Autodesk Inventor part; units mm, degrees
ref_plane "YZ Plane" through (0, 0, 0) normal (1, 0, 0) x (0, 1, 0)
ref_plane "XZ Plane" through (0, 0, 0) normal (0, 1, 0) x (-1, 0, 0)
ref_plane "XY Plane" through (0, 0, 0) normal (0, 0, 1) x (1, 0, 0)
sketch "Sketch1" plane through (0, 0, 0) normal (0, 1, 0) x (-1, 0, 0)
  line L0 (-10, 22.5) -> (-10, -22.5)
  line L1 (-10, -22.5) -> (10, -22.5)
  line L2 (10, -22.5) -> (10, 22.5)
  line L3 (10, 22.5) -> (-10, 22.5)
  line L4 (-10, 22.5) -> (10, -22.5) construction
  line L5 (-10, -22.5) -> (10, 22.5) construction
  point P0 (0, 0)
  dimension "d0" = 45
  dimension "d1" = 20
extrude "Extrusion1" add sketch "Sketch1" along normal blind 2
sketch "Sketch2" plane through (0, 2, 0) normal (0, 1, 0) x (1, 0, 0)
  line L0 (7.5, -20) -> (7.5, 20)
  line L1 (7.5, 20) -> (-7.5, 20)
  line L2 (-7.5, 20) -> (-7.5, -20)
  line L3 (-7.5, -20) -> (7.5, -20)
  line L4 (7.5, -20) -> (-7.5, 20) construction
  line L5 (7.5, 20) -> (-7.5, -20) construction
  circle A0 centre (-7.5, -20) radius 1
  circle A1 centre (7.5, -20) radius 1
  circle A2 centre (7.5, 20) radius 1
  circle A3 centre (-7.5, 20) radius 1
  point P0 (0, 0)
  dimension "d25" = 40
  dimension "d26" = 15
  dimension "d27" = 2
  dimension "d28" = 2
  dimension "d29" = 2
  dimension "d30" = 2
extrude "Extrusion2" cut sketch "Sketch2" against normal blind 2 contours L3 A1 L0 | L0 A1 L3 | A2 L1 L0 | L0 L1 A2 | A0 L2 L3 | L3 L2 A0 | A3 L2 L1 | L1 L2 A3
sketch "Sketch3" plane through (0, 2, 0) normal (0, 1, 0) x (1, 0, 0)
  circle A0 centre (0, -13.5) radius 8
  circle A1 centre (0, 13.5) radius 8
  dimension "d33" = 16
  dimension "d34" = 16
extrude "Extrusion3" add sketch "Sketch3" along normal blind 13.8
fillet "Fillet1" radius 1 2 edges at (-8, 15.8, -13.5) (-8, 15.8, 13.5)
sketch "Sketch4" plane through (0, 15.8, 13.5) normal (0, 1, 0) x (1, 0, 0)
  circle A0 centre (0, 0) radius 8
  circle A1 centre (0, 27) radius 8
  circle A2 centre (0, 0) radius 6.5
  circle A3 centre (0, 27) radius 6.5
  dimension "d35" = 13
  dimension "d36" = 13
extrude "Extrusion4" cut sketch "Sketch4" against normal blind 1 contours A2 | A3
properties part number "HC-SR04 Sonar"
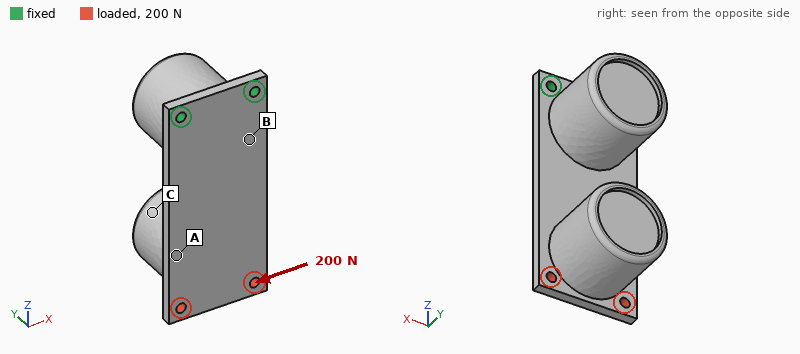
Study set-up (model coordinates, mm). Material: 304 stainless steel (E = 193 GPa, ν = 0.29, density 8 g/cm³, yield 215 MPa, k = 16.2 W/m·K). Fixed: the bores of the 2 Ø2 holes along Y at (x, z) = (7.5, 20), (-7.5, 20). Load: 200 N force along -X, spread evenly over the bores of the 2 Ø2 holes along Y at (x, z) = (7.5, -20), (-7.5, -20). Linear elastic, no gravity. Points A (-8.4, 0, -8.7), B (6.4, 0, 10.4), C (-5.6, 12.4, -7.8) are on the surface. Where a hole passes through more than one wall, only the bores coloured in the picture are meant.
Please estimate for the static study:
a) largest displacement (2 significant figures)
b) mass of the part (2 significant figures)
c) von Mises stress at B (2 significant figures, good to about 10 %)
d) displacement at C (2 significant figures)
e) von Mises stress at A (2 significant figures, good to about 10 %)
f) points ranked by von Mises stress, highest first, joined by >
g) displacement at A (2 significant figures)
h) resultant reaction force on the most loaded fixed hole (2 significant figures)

20 µm
56 g
24 MPa
9.4 µm
14 MPa
B > A > C
12 µm
530 N
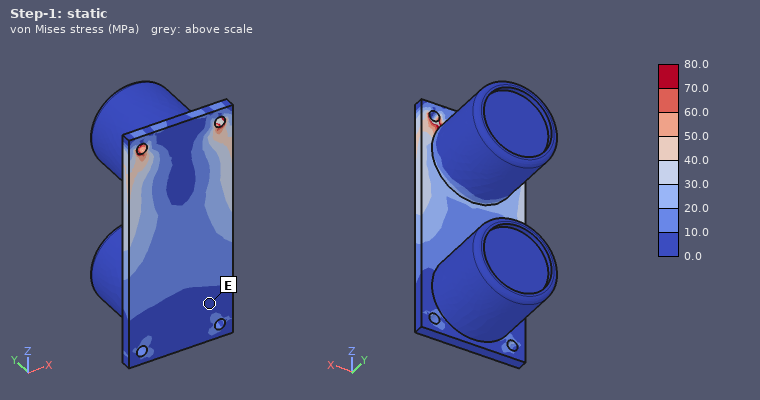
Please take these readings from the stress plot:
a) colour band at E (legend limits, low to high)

0.0 to 10.0 MPa
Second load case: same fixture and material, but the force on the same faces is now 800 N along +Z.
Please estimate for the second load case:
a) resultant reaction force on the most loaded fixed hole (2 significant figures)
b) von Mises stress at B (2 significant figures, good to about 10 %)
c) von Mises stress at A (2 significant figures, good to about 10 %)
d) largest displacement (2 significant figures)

410 N
19 MPa
23 MPa
10 µm
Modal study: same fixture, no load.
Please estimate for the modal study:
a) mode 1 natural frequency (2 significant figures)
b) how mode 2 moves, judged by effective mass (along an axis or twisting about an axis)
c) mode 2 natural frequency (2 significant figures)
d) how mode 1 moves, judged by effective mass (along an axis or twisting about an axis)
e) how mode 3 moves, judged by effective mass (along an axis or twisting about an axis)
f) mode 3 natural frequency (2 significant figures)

600 Hz
along X
2000 Hz
along Y
along Y
2700 Hz
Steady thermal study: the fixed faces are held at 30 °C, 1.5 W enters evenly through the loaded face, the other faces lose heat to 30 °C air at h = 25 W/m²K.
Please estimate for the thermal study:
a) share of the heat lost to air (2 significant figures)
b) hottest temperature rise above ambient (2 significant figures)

73 %
38 K
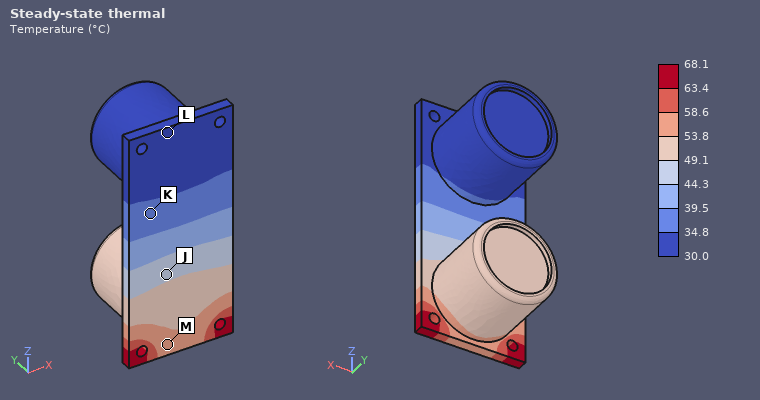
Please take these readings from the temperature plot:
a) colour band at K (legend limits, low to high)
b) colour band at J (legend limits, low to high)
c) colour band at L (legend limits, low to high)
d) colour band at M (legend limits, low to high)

34.8 to 39.5 °C
44.3 to 49.1 °C
30.0 to 34.8 °C
53.8 to 58.6 °C
